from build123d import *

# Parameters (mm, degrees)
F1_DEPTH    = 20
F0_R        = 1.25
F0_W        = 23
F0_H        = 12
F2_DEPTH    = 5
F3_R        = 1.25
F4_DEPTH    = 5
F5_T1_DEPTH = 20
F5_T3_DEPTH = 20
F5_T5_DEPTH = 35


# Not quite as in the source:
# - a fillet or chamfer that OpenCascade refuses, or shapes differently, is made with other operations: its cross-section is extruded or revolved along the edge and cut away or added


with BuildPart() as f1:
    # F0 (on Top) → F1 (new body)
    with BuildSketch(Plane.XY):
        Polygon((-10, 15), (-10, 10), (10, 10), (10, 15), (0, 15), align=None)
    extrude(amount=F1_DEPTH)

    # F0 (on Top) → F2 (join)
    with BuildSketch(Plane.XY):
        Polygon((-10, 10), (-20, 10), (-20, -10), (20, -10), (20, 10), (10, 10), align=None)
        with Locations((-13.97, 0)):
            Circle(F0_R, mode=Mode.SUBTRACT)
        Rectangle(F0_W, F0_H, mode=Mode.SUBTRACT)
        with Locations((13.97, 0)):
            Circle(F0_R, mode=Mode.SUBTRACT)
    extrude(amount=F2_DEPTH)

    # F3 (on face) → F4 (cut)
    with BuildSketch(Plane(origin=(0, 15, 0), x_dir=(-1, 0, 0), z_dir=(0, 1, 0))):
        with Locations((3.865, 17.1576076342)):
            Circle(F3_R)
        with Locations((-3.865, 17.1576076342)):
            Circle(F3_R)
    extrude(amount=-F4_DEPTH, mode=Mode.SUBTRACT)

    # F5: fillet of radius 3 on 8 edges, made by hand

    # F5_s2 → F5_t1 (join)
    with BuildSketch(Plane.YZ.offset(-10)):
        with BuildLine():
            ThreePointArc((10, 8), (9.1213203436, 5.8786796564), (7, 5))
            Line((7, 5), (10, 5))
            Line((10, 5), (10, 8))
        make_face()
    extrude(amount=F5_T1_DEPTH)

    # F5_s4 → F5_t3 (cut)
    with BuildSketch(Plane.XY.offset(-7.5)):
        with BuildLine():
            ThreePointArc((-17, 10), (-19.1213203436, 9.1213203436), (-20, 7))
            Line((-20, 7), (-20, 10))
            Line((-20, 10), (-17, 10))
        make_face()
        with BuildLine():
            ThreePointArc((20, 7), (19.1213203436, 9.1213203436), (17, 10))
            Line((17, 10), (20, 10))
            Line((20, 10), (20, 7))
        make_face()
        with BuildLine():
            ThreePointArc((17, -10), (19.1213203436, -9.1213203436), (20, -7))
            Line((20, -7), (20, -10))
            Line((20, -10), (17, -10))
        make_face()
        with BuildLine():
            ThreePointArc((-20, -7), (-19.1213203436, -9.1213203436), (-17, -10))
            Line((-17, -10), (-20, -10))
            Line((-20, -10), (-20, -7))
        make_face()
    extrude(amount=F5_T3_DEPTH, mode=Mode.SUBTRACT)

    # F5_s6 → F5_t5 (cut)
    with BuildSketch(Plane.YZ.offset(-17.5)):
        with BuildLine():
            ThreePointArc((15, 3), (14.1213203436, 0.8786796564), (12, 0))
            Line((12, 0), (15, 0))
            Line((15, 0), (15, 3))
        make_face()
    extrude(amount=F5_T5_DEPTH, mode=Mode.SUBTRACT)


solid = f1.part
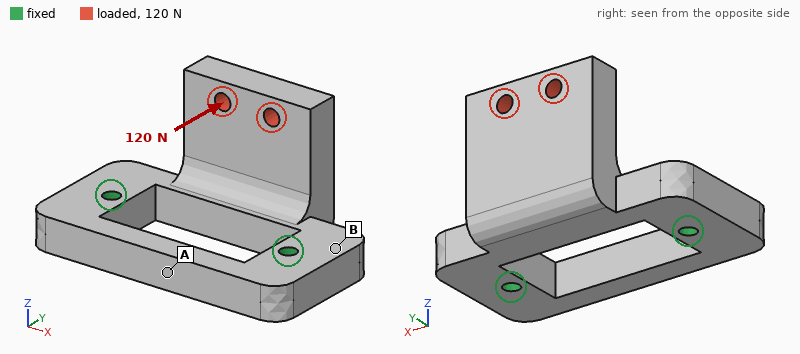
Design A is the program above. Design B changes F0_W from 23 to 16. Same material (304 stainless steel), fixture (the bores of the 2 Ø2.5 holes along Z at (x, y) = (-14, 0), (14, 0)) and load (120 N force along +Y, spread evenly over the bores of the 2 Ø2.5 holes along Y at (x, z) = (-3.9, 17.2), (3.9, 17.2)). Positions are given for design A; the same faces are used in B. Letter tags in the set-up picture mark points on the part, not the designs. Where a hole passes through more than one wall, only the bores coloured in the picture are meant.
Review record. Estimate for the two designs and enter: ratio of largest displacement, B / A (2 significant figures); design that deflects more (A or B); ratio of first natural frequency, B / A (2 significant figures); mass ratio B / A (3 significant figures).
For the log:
0.62
A
1.3
1.09
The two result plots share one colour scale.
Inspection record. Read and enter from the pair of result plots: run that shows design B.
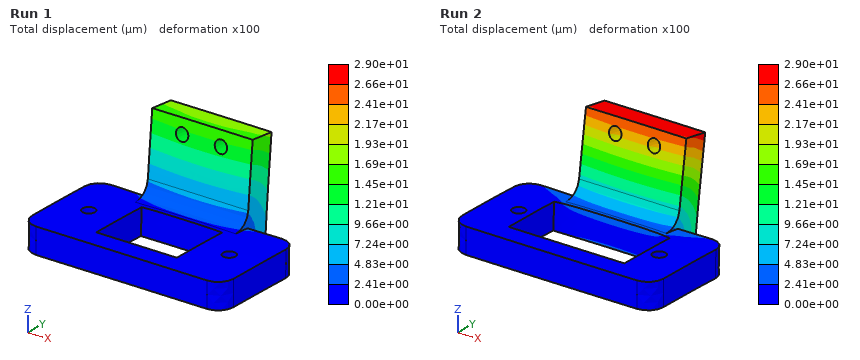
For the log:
Run 1
